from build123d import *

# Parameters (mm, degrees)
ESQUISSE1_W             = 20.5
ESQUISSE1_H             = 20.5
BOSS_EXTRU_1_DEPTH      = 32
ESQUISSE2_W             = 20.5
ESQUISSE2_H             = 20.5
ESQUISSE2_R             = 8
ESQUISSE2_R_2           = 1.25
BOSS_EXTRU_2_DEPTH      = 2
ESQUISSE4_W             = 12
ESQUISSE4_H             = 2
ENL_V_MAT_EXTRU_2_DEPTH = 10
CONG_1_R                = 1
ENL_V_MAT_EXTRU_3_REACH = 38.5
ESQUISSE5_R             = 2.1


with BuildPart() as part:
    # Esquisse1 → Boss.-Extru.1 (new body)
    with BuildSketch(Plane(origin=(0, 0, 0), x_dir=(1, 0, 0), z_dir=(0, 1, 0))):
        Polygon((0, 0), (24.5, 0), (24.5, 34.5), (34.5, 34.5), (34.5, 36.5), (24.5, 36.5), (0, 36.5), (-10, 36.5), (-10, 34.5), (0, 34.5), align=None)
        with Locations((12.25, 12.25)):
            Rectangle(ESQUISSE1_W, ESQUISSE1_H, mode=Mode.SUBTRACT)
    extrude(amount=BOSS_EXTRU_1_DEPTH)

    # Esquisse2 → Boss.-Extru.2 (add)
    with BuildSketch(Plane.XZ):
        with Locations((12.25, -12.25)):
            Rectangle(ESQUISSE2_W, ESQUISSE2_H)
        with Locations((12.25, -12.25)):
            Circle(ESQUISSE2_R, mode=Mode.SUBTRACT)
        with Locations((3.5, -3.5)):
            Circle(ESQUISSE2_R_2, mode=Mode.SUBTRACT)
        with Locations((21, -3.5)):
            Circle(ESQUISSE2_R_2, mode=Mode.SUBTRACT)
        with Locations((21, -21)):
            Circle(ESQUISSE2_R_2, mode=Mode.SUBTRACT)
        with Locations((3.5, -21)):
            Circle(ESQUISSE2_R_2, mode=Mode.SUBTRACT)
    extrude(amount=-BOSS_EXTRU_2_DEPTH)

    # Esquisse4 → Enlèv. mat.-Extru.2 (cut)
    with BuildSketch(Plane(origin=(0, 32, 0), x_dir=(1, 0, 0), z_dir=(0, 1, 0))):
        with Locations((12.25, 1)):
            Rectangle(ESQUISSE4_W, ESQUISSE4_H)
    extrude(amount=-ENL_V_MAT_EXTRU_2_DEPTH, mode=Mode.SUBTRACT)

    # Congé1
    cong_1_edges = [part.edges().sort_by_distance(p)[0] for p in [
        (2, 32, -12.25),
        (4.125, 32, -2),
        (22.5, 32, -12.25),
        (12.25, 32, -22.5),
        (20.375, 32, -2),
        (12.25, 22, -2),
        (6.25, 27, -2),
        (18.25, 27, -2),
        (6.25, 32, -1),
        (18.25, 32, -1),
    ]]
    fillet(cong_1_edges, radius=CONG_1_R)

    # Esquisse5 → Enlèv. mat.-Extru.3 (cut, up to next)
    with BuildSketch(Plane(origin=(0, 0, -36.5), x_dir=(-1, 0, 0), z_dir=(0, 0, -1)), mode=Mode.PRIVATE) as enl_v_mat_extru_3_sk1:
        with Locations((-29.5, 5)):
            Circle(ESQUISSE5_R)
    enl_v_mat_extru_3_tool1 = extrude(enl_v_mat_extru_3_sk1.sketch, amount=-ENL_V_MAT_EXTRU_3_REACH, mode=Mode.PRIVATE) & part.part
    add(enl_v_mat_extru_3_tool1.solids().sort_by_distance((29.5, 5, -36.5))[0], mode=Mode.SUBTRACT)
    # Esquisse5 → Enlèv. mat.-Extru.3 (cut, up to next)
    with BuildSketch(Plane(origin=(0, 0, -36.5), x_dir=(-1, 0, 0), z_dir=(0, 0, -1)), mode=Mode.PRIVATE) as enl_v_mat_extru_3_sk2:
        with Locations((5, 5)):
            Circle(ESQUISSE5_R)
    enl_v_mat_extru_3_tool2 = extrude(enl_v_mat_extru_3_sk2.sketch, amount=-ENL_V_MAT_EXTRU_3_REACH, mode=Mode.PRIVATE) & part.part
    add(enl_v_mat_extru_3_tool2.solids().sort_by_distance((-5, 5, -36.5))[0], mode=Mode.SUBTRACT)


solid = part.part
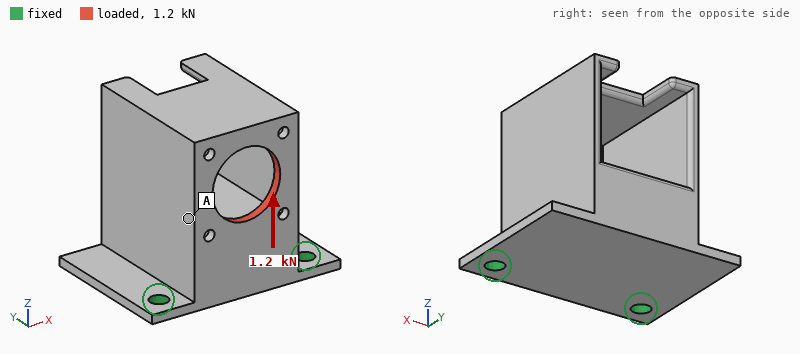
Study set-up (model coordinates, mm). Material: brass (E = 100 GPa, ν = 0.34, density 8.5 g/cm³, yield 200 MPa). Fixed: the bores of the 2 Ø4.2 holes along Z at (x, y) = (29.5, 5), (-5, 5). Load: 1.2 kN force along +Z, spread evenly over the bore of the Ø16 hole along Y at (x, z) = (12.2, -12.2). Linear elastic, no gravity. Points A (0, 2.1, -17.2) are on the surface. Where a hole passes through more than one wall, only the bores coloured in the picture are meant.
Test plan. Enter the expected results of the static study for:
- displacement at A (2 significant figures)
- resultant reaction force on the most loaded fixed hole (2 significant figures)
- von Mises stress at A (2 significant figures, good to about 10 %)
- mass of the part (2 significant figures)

0.095 mm
680 N
21 MPa
140 g
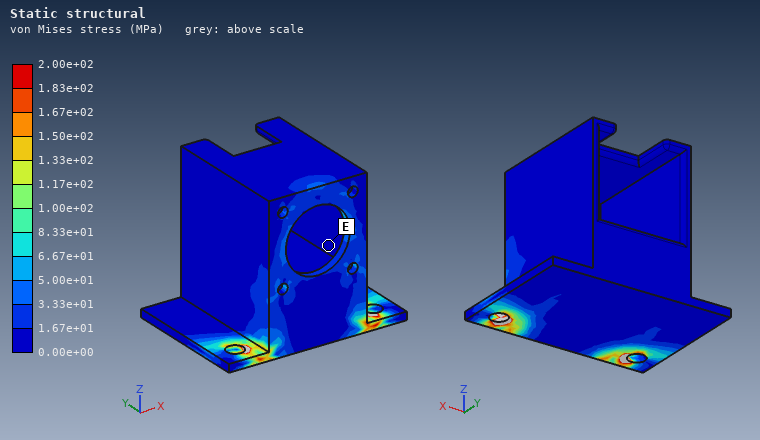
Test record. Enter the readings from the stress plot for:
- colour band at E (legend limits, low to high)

0.00e+00 to 1.67e+01 MPa
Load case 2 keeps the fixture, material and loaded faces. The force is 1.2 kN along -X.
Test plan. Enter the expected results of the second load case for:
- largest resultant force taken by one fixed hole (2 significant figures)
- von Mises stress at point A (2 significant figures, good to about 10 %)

1.2 kN
57 MPa
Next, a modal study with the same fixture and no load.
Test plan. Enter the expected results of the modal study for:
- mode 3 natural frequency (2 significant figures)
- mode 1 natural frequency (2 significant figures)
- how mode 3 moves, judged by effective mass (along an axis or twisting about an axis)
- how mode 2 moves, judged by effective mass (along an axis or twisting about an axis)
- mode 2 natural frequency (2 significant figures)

4800 Hz
690 Hz
along Z
along X
2600 Hz
